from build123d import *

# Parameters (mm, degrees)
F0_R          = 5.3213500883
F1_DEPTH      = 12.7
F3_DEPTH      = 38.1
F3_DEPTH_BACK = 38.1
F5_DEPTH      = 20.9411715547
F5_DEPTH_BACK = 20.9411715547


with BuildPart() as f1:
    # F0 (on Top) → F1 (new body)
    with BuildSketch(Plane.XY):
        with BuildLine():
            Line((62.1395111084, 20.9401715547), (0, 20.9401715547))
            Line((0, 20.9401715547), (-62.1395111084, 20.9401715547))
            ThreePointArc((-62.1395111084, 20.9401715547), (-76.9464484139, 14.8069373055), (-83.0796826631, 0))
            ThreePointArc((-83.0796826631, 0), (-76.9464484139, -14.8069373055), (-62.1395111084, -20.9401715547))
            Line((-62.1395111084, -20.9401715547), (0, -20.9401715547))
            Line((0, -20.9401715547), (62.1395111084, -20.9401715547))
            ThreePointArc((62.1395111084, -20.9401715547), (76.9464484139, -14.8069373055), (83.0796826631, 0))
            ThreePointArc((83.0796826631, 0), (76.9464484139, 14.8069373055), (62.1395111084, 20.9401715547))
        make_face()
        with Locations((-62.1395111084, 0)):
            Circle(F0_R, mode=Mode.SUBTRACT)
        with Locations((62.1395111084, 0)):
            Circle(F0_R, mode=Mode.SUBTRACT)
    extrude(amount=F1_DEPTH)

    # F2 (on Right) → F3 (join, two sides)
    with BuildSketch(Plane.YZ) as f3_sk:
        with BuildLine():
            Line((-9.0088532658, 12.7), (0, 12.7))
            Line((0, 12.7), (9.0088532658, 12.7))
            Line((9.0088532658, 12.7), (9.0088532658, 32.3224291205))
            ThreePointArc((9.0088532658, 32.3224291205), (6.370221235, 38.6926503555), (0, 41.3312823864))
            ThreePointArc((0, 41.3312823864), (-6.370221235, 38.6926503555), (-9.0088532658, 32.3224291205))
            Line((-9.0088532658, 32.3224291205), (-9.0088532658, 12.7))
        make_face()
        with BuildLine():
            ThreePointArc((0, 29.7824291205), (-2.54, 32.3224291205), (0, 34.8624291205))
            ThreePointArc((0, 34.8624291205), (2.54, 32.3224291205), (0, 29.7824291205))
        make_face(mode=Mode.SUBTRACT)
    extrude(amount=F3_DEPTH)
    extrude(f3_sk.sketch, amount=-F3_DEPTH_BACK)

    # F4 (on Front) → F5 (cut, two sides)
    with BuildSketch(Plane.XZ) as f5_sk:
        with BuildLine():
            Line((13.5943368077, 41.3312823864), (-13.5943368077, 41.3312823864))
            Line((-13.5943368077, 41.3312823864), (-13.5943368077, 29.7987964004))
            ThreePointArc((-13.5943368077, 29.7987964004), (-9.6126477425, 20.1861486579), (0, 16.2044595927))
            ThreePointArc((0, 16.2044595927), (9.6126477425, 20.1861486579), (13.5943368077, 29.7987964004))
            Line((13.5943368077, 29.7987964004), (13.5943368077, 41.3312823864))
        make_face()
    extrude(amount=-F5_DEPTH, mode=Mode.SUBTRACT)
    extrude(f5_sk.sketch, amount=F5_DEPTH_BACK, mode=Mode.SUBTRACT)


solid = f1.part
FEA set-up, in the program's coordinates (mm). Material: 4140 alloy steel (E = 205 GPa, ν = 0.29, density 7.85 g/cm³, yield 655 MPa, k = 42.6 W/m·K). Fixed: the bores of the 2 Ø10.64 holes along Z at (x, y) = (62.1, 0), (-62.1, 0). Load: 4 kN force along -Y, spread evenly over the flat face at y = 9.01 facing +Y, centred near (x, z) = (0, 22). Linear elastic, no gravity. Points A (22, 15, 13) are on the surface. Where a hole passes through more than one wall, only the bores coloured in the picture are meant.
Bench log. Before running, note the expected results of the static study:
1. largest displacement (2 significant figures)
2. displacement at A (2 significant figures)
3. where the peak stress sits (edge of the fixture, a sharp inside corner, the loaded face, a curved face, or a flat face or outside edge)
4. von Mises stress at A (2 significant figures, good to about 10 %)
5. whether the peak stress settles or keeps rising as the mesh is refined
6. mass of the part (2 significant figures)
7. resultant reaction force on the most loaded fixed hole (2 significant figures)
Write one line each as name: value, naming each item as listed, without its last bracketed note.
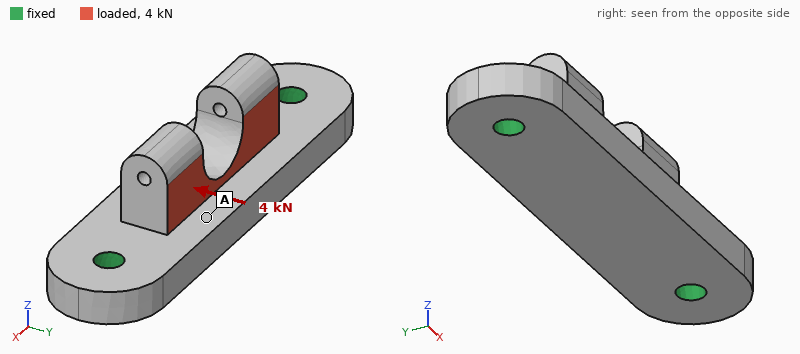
largest displacement: 23 µm
displacement at A: 10 µm
where the peak stress sits: edge of the fixture
von Mises stress at A: 8.3 MPa
whether the peak stress settles or keeps rising as the mesh is refined: keeps rising
mass of the part: 840 g
resultant reaction force on the most loaded fixed hole: 2.0 kN
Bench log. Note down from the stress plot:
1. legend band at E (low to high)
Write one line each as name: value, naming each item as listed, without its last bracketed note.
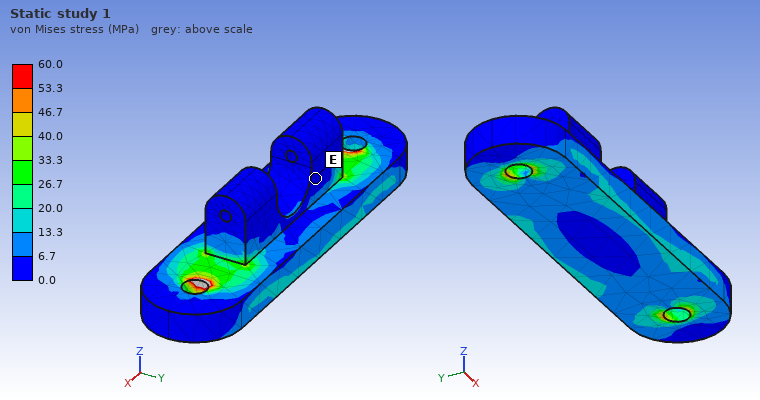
legend band at E: 0.0 to 6.7 MPa
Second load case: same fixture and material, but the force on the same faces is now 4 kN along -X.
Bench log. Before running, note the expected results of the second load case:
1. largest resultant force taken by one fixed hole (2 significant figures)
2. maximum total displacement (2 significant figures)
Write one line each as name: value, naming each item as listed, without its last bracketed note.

largest resultant force taken by one fixed hole: 2.1 kN
maximum total displacement: 3.5 µm
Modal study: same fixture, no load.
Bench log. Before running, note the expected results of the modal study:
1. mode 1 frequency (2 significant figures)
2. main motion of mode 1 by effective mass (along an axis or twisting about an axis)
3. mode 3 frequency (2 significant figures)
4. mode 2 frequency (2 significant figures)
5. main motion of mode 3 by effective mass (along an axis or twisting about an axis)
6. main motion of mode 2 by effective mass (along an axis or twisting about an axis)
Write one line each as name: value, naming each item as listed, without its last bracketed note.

mode 1 frequency: 3900 Hz
main motion of mode 1 by effective mass: along Z
mode 3 frequency: 6900 Hz
mode 2 frequency: 4400 Hz
main motion of mode 3 by effective mass: along Y
main motion of mode 2 by effective mass: along Y
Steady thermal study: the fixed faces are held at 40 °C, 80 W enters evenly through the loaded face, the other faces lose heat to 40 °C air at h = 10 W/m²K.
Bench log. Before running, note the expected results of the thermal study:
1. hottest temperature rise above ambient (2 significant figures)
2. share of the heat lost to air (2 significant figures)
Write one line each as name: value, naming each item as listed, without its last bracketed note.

hottest temperature rise above ambient: 82 K
share of the heat lost to air: 11 %
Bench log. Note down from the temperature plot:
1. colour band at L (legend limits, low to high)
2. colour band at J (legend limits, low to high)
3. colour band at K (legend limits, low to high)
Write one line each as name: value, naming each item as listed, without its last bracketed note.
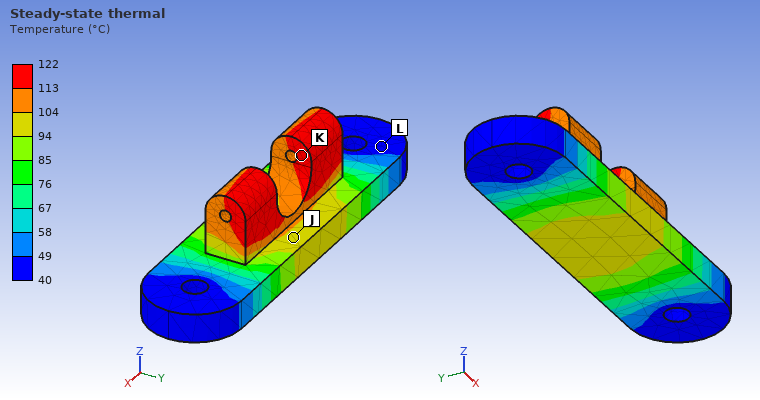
colour band at L: 40 to 49 °C
colour band at J: 94 to 104 °C
colour band at K: 113 to 122 °C
